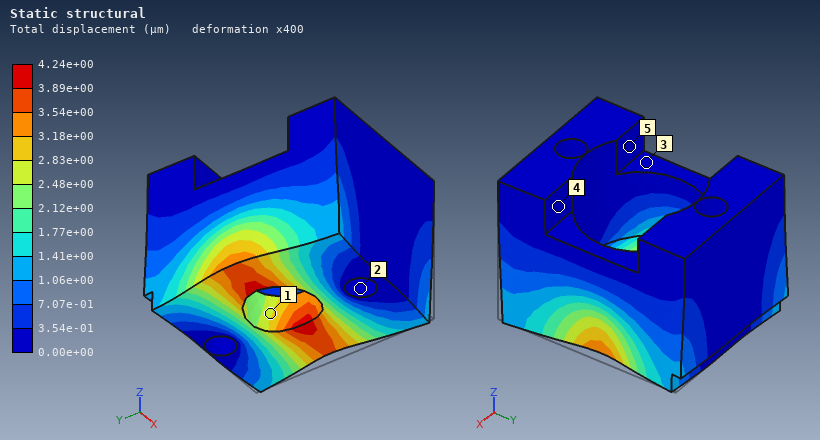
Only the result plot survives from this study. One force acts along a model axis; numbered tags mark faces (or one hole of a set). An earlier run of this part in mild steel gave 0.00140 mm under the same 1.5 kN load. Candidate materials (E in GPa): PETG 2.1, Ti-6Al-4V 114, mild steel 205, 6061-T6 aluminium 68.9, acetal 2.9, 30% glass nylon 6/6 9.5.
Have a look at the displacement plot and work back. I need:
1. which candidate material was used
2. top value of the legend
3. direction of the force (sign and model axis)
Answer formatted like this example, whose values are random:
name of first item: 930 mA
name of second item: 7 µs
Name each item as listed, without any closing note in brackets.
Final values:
which candidate material was used: 6061-T6 aluminium
top value of the legend: 4.24e+00 µm
direction of the force: -X
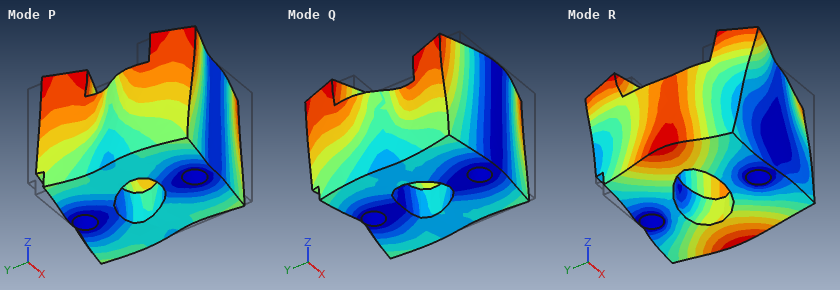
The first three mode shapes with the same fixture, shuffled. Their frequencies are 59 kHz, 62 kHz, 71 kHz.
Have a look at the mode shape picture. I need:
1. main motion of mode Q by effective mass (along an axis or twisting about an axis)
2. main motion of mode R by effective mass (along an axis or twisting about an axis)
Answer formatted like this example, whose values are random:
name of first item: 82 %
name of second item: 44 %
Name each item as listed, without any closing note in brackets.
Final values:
main motion of mode Q by effective mass: along Y
main motion of mode R by effective mass: twisting about Y
